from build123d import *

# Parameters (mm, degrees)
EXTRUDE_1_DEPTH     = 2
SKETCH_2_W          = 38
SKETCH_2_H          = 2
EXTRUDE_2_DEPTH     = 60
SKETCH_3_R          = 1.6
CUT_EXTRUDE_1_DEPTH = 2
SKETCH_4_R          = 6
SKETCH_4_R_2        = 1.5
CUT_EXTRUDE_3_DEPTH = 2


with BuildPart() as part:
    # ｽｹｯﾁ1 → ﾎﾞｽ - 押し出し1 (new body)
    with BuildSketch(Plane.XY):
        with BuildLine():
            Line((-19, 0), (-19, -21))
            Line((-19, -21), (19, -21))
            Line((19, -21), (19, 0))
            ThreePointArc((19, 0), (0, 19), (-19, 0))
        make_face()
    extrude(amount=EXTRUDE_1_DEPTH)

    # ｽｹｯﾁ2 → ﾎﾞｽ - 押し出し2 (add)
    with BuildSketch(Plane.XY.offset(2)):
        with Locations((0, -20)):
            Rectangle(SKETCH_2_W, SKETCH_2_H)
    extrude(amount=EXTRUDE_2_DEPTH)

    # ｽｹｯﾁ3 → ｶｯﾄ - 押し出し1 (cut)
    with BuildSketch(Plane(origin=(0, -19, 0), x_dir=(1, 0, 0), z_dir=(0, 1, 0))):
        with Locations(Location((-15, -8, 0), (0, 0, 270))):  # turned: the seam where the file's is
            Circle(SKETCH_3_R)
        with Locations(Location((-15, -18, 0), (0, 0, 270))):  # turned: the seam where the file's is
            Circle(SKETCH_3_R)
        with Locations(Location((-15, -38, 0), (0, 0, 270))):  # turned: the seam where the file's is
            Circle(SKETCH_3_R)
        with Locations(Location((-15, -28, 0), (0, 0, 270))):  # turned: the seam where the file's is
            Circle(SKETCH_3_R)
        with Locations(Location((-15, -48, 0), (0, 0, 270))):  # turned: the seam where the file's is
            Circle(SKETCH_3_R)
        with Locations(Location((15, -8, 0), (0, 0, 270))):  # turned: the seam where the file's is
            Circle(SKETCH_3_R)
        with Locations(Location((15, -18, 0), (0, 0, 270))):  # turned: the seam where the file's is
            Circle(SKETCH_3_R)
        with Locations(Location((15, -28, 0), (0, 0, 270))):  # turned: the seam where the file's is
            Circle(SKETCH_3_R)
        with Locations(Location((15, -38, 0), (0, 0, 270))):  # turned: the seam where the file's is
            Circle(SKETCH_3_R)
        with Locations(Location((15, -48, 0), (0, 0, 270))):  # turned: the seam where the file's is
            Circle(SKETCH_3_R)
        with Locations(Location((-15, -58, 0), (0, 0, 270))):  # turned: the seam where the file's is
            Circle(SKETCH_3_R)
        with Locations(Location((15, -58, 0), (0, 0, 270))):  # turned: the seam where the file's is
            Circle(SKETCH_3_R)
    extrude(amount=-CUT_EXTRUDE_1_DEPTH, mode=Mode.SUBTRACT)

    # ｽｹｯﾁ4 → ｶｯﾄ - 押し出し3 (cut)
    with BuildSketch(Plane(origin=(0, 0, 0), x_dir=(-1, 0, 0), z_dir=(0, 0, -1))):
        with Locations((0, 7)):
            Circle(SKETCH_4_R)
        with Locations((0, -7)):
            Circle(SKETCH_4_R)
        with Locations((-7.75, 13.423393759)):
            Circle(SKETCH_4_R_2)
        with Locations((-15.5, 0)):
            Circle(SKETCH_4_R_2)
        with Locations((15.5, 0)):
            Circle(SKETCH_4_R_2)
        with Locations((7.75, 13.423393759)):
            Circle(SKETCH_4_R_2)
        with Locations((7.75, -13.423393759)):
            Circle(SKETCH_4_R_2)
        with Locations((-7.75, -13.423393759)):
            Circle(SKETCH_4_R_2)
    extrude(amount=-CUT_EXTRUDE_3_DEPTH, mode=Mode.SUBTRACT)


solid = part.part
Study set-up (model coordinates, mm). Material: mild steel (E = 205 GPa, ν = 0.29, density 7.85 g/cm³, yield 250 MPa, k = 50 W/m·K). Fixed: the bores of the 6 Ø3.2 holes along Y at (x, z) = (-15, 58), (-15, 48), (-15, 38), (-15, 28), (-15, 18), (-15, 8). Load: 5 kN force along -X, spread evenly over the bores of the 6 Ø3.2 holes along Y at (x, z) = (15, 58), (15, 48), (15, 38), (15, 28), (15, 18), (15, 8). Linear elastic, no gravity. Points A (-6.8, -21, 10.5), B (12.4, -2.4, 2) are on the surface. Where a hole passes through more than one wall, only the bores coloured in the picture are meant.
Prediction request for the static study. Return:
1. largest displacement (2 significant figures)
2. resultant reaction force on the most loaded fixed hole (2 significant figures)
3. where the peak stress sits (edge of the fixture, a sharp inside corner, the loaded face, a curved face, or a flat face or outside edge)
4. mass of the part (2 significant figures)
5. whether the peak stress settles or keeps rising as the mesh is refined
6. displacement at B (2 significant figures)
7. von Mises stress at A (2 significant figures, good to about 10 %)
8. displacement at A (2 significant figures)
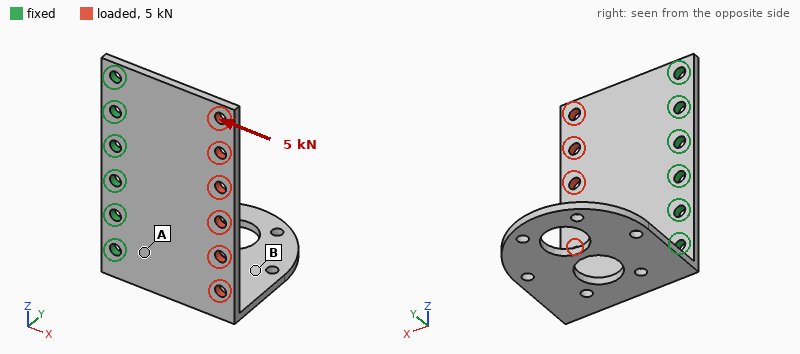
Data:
8.2 µm
970 N
edge of the fixture
51 g
keeps rising
2.8 µm
41 MPa
1.8 µm
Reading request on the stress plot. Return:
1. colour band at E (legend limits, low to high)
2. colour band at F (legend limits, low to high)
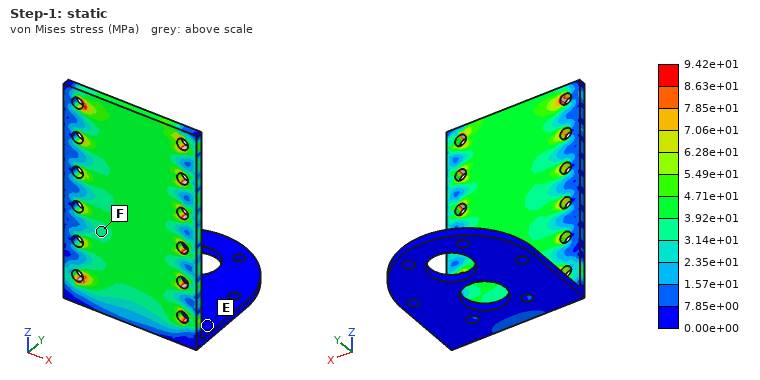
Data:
0.00e+00 to 7.85e+00 MPa
3.14e+01 to 3.92e+01 MPa
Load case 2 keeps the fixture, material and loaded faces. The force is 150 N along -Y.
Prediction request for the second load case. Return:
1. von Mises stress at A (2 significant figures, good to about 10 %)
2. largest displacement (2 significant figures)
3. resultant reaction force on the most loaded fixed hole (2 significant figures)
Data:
35 MPa
0.16 mm
34 N
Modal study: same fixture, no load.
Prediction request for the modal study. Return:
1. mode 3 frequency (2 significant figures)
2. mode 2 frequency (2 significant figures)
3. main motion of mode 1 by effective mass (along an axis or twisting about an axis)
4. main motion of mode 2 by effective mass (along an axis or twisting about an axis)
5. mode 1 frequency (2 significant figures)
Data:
2000 Hz
1200 Hz
along Z
along Y
890 Hz
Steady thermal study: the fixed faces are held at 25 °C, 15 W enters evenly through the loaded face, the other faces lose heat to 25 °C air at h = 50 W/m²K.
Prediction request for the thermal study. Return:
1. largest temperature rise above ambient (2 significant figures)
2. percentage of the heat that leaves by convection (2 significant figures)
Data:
58 K
44 %
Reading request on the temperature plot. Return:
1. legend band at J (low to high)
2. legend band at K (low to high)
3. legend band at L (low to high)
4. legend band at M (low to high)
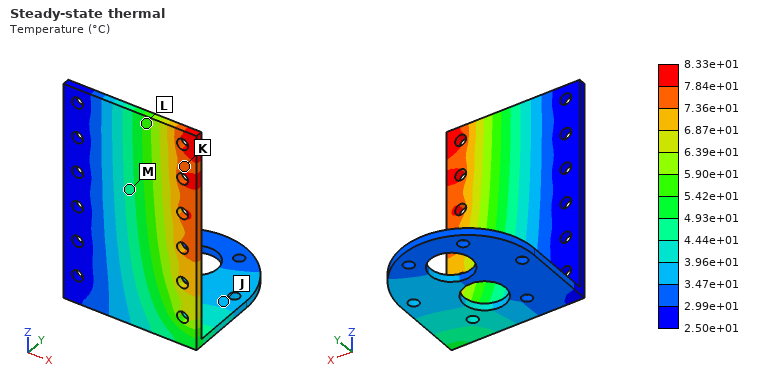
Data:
3.47e+01 to 3.96e+01 °C
7.36e+01 to 7.84e+01 °C
5.42e+01 to 5.90e+01 °C
4.44e+01 to 4.93e+01 °C
